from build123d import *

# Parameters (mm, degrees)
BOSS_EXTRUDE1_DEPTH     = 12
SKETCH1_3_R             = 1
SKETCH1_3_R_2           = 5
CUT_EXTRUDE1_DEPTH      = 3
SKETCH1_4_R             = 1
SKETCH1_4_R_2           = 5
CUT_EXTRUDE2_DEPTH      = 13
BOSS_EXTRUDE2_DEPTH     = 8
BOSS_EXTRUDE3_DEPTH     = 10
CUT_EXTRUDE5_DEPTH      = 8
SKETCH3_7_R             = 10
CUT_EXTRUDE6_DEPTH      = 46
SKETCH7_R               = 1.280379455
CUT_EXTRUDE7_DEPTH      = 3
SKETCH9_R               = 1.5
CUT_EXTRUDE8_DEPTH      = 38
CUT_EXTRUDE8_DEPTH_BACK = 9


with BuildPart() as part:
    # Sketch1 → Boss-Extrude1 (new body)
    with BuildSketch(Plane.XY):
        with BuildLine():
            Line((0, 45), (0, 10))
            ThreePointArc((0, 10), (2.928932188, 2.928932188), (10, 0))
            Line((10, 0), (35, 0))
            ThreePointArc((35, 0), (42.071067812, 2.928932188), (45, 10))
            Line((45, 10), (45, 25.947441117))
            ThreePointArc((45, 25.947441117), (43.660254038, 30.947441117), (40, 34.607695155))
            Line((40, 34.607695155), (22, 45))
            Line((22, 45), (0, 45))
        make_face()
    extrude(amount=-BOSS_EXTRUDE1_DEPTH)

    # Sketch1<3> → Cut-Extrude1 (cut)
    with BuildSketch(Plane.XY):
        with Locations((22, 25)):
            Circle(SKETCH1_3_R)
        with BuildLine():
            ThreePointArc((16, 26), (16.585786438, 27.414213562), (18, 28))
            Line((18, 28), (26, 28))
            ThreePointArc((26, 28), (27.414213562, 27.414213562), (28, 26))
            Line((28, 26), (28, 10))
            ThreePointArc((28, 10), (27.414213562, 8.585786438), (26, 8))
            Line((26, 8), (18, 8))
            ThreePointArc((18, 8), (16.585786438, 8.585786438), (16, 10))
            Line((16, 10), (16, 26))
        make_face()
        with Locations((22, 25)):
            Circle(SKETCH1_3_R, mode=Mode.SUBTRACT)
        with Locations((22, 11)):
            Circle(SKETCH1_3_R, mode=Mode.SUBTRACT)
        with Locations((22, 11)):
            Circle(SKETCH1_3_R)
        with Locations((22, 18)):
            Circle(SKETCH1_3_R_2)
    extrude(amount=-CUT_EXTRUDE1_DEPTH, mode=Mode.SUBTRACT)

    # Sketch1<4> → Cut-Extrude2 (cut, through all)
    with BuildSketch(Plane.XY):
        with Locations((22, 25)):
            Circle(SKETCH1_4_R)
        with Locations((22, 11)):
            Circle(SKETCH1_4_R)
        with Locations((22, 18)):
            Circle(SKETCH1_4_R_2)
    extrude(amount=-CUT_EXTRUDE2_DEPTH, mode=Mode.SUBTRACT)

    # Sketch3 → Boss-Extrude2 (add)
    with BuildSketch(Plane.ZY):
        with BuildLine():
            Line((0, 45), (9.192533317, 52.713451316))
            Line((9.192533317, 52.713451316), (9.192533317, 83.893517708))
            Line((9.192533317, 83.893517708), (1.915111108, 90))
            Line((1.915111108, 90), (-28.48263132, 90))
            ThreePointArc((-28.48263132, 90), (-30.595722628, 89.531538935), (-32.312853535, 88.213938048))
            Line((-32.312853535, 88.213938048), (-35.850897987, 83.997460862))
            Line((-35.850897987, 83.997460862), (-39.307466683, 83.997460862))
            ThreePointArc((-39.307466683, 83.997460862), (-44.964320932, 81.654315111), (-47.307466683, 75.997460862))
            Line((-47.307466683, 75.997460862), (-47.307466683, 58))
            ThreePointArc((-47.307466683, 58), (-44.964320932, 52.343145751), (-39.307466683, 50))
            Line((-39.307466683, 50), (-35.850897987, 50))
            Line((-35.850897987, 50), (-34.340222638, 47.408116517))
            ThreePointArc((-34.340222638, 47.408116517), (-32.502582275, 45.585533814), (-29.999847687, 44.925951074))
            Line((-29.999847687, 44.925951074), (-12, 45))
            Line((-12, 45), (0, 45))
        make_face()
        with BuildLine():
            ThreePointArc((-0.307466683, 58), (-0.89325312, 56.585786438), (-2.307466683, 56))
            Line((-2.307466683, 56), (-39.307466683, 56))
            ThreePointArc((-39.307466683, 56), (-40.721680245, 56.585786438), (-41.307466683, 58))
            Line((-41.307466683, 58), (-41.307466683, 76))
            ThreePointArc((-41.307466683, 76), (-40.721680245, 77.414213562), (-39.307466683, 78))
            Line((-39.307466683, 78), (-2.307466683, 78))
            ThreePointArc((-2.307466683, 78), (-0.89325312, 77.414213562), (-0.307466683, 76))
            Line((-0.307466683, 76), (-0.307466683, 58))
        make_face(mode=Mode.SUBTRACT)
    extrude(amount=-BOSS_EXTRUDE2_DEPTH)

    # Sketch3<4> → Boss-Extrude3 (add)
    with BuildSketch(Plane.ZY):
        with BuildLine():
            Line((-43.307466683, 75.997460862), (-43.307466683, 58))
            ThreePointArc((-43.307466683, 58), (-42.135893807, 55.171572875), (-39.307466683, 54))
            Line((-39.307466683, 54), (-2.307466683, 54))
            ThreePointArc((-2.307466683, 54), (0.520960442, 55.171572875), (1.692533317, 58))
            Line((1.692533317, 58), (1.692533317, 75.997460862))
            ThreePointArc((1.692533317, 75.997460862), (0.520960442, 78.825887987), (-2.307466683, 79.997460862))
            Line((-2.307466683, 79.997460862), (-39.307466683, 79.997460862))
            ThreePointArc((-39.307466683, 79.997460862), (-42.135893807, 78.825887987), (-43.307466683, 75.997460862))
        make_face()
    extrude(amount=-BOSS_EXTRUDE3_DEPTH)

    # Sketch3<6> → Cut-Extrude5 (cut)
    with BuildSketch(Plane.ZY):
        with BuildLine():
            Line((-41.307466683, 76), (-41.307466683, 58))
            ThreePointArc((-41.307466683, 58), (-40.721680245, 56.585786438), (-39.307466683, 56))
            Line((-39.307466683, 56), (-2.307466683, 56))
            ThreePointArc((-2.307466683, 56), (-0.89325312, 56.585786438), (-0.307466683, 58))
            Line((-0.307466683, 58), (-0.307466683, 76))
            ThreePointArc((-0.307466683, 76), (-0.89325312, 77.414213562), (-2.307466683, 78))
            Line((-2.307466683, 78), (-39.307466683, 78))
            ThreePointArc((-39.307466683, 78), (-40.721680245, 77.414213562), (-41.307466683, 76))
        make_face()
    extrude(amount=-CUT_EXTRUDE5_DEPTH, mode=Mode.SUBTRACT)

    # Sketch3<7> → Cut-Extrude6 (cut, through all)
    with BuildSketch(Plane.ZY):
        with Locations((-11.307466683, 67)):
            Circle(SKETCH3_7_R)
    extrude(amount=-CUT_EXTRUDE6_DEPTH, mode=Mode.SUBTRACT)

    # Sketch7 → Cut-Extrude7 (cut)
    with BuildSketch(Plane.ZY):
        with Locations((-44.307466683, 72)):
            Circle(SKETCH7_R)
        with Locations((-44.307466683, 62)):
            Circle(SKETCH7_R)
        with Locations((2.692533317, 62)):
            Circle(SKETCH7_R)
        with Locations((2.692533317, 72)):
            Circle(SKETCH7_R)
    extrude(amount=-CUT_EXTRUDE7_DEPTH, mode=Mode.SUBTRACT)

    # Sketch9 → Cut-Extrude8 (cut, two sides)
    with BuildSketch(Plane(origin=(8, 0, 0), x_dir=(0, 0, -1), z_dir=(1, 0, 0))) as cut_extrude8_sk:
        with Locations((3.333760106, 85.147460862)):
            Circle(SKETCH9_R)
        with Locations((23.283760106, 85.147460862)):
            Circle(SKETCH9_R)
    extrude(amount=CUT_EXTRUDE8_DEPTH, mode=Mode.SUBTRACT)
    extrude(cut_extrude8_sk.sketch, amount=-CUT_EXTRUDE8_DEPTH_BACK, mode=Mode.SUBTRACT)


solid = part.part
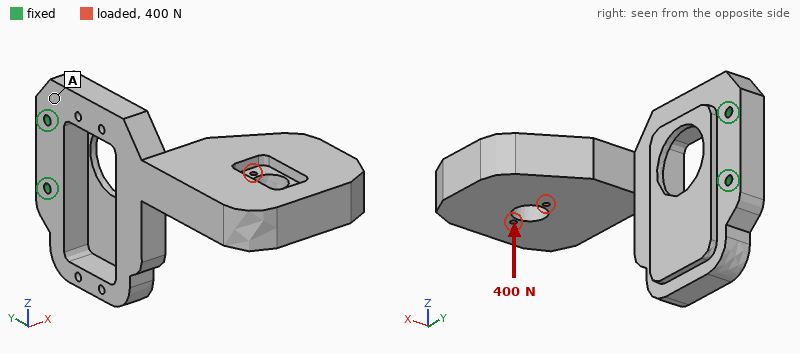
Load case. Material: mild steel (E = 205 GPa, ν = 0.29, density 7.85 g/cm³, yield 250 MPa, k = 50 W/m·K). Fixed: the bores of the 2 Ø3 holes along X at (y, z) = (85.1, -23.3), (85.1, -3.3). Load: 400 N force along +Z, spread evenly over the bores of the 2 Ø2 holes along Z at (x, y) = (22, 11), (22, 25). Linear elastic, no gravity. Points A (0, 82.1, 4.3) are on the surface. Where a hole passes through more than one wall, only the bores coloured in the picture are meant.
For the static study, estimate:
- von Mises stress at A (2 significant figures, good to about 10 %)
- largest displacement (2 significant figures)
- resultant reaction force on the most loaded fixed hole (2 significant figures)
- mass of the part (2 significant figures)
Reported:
16 MPa
0.10 mm
1.1 kN
260 g
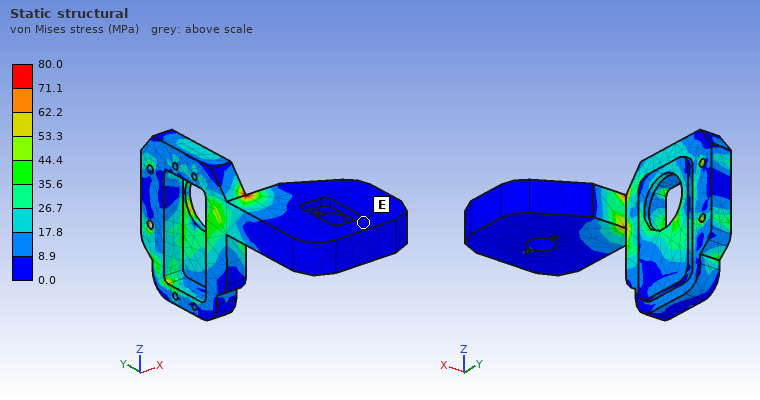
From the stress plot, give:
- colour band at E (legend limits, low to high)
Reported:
0.0 to 8.9 MPa
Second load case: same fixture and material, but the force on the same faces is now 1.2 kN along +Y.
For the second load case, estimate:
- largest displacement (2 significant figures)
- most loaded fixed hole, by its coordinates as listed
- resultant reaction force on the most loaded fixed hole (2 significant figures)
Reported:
0.47 mm
(85.1, -3.3)
870 N
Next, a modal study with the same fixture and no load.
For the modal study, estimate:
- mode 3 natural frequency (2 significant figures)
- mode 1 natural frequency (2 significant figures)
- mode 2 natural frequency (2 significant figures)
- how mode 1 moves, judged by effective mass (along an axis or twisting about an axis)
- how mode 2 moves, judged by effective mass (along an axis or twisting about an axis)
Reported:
2200 Hz
440 Hz
1000 Hz
along X
along Z
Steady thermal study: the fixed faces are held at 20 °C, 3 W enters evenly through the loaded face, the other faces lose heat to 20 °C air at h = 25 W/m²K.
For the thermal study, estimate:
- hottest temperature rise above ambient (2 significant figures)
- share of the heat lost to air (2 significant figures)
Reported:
13 K
65 %
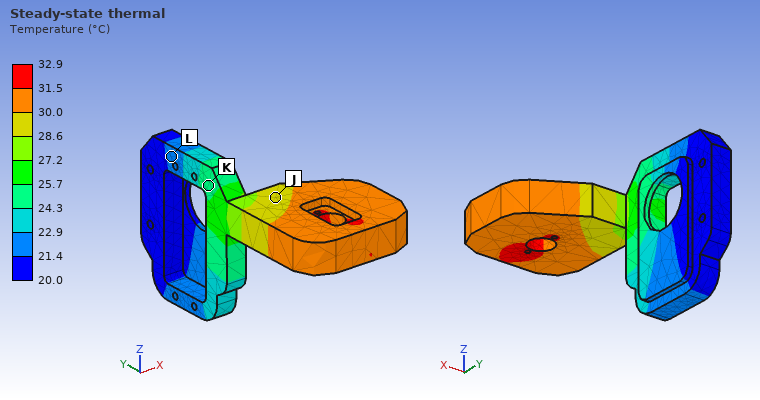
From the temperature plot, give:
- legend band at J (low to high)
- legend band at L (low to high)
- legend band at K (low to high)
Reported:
28.6 to 30.0 °C
21.4 to 22.9 °C
24.3 to 25.7 °C
